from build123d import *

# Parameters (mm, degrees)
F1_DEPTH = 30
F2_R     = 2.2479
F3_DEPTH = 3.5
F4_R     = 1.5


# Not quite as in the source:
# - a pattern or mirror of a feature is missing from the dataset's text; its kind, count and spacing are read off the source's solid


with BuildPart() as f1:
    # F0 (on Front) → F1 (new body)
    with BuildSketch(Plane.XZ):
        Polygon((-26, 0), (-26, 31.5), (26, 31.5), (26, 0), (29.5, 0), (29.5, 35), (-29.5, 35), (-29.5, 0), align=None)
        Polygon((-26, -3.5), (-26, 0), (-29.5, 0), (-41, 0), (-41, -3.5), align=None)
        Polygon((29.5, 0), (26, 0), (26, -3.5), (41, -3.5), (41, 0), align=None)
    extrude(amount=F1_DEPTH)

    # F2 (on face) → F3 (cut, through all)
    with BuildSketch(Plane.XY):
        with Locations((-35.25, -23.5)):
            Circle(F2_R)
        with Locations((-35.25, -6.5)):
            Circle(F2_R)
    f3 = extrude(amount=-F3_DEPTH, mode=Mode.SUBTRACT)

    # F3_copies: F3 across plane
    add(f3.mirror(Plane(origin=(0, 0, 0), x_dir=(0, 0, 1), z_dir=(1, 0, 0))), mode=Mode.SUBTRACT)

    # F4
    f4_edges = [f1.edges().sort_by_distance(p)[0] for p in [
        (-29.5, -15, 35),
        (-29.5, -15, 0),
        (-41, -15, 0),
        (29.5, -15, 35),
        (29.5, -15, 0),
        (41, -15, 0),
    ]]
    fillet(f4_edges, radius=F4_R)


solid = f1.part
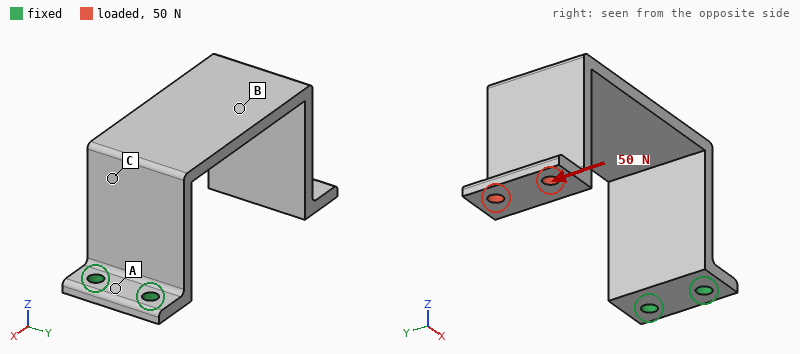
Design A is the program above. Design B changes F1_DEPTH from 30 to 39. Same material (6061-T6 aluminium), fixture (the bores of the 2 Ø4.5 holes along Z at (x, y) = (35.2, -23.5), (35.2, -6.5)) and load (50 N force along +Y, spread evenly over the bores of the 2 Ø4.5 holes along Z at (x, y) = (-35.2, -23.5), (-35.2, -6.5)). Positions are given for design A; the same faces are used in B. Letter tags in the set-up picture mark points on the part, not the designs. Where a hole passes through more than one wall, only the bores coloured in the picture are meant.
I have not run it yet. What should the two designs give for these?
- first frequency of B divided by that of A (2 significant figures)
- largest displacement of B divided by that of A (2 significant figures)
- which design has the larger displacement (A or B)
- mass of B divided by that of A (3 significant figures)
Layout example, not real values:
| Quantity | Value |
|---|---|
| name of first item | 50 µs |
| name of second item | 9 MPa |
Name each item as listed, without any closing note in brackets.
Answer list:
| Quantity | Value |
|---|---|
| first frequency of B divided by that of A | 0.99 |
| largest displacement of B divided by that of A | 0.74 |
| which design has the larger displacement | A |
| mass of B divided by that of A | 1.30 |
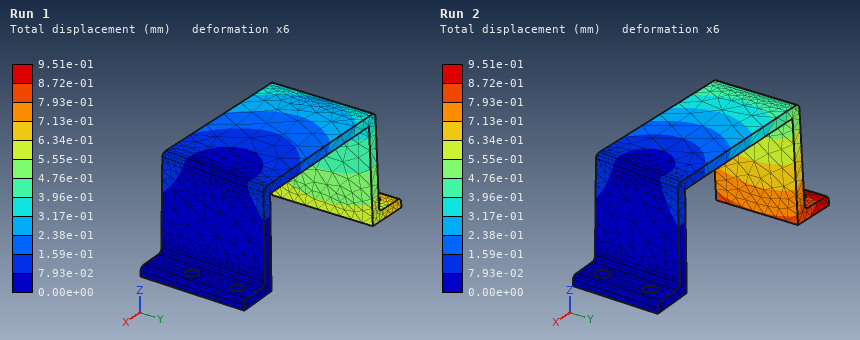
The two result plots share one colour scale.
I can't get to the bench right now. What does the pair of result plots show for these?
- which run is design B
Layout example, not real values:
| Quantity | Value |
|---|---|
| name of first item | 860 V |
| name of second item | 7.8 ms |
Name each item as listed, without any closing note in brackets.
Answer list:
| Quantity | Value |
|---|---|
| which run is design B | Run 1 |
